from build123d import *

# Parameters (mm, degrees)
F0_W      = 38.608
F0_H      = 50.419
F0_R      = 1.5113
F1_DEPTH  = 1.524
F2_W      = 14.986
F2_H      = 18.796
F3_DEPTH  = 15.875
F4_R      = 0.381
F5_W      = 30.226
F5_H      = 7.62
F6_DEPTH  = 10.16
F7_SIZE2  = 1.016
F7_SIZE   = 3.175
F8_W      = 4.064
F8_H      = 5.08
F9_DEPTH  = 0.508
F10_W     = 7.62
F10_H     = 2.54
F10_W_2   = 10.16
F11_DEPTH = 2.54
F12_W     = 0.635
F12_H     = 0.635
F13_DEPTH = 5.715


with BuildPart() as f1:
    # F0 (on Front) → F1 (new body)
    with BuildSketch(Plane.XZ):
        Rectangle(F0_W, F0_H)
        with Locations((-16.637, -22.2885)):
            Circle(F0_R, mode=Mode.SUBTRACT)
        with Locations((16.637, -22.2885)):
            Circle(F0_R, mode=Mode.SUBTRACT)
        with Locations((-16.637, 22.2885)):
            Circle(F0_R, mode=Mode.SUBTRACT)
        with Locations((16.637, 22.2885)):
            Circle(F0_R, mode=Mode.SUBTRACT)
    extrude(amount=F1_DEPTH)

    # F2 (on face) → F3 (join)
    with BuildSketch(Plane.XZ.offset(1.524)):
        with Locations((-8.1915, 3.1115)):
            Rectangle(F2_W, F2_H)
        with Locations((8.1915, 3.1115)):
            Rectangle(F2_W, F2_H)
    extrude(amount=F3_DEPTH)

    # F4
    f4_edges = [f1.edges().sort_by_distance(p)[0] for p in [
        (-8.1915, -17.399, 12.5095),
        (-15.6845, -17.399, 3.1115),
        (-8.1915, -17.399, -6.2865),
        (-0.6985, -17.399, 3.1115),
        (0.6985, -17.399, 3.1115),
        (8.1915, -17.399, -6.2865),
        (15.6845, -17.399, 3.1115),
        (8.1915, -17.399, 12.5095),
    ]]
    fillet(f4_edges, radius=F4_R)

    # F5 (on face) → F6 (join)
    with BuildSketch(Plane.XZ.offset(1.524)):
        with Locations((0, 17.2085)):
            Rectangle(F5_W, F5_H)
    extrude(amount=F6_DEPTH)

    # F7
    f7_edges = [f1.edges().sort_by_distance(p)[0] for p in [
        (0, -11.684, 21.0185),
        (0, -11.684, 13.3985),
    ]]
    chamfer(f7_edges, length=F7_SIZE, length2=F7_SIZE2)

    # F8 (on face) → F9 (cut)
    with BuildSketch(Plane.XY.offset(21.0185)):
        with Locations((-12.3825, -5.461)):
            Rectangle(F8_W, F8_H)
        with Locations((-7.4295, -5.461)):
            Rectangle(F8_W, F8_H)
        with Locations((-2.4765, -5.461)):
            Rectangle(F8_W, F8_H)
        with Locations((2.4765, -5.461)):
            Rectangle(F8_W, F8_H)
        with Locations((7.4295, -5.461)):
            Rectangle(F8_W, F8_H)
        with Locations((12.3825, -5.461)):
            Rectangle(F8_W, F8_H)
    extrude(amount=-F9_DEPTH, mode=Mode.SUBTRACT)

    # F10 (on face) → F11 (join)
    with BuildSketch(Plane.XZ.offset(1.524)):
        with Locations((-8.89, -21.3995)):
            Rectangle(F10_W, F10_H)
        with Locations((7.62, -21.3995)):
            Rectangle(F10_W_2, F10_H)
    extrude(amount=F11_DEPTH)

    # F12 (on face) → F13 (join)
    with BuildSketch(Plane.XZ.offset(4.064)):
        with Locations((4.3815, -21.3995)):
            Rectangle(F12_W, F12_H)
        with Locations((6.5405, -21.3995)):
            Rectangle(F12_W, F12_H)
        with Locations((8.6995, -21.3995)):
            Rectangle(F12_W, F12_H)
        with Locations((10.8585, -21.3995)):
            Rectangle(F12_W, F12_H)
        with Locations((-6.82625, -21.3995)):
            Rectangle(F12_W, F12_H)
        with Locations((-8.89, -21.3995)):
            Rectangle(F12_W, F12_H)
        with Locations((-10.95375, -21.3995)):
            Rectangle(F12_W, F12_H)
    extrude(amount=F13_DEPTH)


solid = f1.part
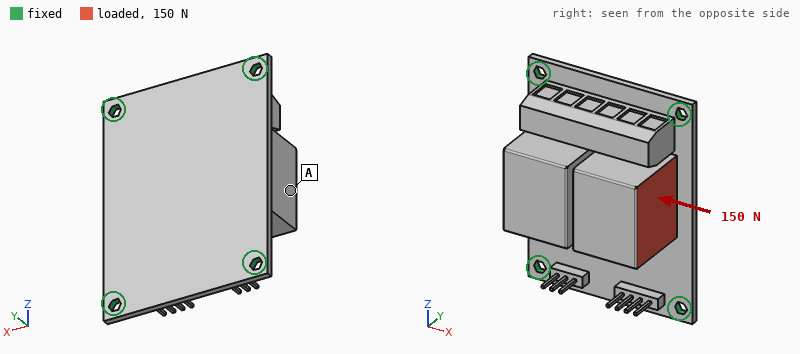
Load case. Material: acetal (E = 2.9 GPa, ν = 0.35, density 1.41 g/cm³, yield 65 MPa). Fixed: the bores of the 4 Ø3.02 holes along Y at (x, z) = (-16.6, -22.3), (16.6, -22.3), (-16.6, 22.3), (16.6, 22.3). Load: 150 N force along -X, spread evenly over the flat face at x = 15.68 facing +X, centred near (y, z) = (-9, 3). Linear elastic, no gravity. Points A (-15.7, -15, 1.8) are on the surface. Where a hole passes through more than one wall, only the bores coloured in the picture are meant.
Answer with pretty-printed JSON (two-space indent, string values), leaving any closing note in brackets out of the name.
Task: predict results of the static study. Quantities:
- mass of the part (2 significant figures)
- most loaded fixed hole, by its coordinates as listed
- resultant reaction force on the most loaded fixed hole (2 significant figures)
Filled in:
{
  "mass of the part": "20 g",
  "most loaded fixed hole, by its coordinates as listed": "(-16.6, 22.3)",
  "resultant reaction force on the most loaded fixed hole": "85 N"
}
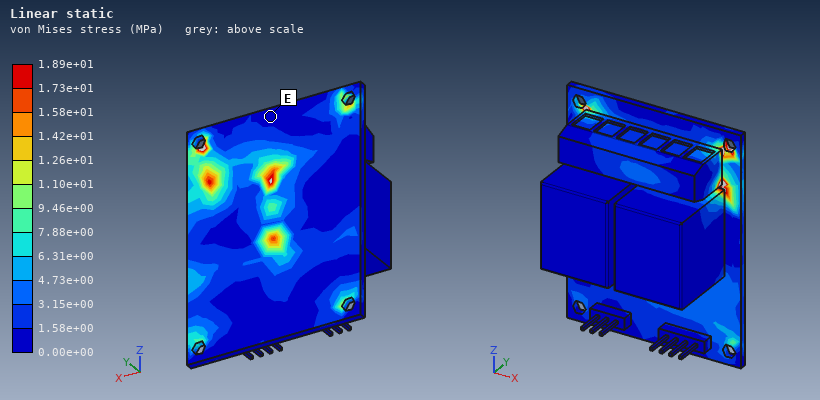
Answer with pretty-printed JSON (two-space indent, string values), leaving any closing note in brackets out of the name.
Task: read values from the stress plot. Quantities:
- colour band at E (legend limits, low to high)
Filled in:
{
  "colour band at E": "0.00e+00 to 1.58e+00 MPa"
}
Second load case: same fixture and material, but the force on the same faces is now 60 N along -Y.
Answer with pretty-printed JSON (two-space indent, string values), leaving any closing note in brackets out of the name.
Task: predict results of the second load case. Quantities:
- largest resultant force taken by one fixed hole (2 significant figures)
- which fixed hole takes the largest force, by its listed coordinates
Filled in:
{
  "largest resultant force taken by one fixed hole": "50 N",
  "which fixed hole takes the largest force, by its listed coordinates": "(16.6, 22.3)"
}
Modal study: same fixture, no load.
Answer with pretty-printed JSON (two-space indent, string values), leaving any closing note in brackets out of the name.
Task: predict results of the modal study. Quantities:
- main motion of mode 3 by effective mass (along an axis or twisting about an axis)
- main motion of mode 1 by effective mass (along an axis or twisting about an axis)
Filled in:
{
  "main motion of mode 3 by effective mass": "along X",
  "main motion of mode 1 by effective mass": "along Y"
}
